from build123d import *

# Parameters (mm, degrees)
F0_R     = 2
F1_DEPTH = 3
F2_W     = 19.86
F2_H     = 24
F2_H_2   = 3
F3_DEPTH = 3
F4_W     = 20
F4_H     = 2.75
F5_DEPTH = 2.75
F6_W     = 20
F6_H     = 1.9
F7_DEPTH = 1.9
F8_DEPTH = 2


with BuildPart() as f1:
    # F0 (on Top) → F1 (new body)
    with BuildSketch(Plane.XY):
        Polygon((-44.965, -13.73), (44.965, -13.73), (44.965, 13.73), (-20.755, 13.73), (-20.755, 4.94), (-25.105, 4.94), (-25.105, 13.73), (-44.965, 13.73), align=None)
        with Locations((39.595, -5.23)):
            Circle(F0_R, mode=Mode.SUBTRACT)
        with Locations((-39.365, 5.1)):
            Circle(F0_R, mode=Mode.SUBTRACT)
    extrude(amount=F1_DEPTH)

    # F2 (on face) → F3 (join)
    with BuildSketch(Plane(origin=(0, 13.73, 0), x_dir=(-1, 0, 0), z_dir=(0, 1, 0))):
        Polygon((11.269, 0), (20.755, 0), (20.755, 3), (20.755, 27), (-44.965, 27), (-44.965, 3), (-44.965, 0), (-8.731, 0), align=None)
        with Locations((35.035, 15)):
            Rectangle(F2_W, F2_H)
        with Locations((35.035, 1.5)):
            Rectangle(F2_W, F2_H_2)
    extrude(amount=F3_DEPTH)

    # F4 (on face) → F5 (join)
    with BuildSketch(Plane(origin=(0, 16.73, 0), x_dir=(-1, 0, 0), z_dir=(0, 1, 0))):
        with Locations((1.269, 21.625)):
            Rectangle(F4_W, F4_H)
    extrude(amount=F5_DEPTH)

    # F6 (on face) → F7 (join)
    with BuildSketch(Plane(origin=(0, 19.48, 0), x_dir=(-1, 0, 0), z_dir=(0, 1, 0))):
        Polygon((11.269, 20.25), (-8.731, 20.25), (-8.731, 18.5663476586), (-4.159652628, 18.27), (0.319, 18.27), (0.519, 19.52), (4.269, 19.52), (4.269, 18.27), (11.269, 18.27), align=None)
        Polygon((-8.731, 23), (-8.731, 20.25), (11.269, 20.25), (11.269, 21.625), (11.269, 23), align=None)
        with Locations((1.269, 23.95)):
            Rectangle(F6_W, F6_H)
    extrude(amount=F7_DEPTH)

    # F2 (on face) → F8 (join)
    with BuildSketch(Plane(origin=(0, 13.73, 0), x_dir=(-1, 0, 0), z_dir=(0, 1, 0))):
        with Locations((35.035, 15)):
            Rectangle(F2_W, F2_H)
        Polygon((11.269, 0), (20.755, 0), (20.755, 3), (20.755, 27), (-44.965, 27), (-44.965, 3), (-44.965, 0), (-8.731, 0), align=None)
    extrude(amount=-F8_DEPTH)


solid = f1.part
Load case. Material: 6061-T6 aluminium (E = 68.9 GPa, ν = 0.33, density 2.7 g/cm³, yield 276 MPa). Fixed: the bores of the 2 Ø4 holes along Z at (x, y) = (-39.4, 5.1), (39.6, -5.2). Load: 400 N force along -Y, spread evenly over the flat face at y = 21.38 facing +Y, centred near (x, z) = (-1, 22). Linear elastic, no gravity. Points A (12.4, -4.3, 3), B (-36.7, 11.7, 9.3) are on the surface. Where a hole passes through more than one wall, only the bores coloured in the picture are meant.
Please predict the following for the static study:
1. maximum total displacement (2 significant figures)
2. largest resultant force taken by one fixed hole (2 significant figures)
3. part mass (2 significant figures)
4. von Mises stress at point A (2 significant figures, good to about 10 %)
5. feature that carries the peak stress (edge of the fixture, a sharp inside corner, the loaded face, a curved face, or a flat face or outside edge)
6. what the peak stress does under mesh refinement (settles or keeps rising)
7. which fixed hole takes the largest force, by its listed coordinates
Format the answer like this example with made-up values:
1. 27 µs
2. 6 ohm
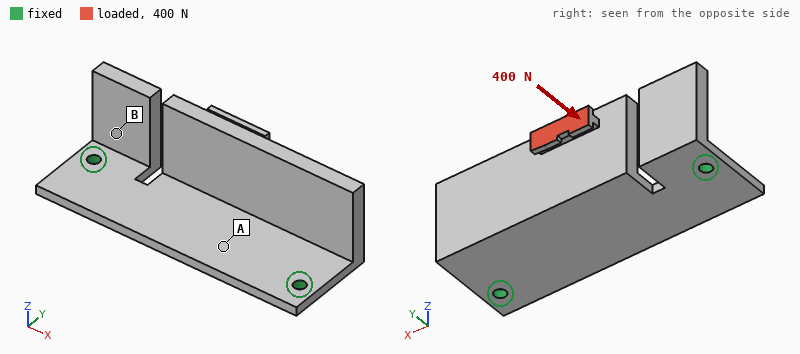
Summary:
1. 0.74 mm
2. 220 N
3. 50 g
4. 43 MPa
5. edge of the fixture
6. keeps rising
7. (-39.4, 5.1)
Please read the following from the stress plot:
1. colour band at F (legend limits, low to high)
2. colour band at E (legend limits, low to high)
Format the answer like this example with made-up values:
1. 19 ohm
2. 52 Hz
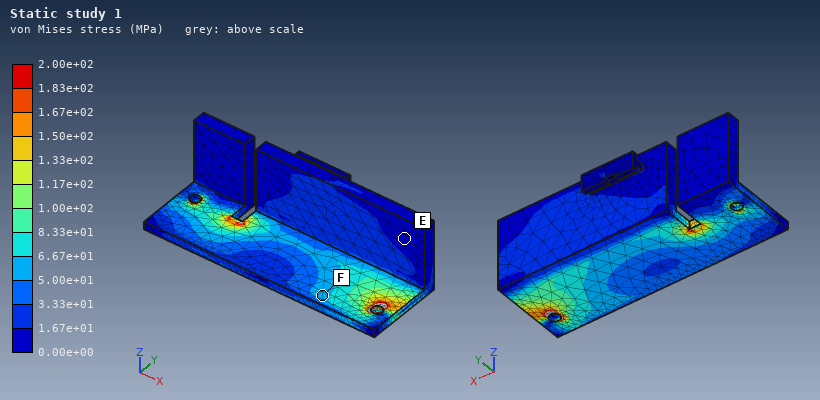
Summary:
1. 5.00e+01 to 6.67e+01 MPa
2. 0.00e+00 to 1.67e+01 MPa
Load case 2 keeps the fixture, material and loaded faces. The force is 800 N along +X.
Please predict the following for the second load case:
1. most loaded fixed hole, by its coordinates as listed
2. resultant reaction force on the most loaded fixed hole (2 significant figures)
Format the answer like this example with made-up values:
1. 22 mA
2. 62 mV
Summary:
1. (39.6, -5.2)
2. 740 N
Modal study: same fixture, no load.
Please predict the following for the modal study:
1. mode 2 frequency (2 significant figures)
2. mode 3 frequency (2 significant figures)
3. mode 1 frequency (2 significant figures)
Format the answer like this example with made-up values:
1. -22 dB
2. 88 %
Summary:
1. 2000 Hz
2. 2300 Hz
3. 960 Hz
